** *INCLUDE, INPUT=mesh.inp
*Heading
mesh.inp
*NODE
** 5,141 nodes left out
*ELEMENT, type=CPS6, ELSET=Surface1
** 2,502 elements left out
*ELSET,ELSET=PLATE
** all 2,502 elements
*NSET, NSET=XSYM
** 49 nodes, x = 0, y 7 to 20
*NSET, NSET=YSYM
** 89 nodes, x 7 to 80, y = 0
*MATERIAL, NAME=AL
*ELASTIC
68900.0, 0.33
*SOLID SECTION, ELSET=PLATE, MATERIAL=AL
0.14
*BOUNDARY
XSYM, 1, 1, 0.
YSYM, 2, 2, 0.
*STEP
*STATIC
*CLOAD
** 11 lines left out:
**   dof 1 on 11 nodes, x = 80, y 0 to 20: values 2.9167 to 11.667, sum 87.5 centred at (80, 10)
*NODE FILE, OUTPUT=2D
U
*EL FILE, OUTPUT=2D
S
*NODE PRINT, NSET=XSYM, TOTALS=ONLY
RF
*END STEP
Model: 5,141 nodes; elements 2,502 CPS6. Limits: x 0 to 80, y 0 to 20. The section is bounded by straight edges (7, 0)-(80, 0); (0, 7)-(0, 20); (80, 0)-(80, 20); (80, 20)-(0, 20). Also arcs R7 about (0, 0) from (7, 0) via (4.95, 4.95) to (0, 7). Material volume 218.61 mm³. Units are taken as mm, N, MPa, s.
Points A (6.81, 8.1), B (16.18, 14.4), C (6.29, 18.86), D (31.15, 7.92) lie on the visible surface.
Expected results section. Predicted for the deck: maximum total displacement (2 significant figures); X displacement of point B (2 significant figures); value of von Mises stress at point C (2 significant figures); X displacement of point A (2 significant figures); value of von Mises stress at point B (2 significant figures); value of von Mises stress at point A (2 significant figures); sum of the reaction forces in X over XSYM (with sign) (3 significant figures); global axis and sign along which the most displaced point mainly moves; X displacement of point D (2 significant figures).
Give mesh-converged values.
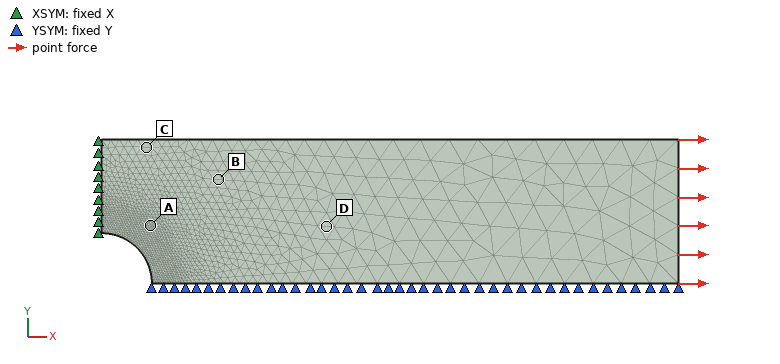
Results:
0.041 mm
0.0095 mm
36 MPa
0.0059 mm
38 MPa
48 MPa
-87.5 N
+X
0.017 mm
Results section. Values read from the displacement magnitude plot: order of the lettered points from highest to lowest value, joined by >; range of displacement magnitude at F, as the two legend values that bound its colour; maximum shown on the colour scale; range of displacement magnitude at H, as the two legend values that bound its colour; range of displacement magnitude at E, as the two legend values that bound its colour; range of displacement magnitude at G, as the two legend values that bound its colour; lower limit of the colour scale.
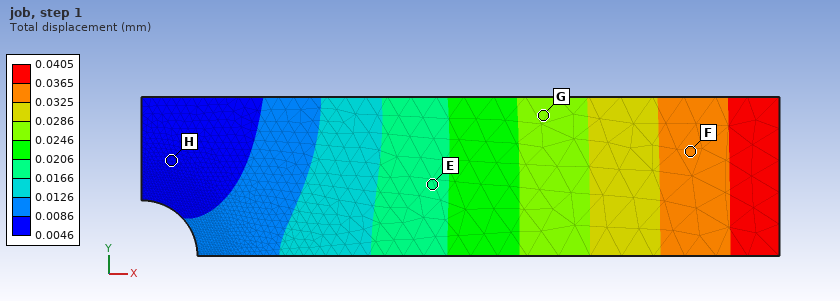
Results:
F > G > E > H
0.0325 to 0.0365 mm
0.0405 mm
0.0046 to 0.0086 mm
0.0166 to 0.0206 mm
0.0246 to 0.0286 mm
0.0046 mm
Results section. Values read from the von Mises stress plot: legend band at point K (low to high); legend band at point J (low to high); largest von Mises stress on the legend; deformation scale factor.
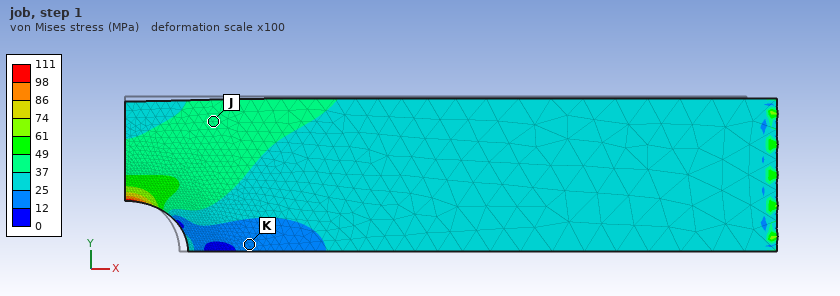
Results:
12 to 25 MPa
37 to 49 MPa
111 MPa
100
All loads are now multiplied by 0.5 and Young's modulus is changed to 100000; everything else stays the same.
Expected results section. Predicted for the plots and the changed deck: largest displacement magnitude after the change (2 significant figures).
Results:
0.014 mm
